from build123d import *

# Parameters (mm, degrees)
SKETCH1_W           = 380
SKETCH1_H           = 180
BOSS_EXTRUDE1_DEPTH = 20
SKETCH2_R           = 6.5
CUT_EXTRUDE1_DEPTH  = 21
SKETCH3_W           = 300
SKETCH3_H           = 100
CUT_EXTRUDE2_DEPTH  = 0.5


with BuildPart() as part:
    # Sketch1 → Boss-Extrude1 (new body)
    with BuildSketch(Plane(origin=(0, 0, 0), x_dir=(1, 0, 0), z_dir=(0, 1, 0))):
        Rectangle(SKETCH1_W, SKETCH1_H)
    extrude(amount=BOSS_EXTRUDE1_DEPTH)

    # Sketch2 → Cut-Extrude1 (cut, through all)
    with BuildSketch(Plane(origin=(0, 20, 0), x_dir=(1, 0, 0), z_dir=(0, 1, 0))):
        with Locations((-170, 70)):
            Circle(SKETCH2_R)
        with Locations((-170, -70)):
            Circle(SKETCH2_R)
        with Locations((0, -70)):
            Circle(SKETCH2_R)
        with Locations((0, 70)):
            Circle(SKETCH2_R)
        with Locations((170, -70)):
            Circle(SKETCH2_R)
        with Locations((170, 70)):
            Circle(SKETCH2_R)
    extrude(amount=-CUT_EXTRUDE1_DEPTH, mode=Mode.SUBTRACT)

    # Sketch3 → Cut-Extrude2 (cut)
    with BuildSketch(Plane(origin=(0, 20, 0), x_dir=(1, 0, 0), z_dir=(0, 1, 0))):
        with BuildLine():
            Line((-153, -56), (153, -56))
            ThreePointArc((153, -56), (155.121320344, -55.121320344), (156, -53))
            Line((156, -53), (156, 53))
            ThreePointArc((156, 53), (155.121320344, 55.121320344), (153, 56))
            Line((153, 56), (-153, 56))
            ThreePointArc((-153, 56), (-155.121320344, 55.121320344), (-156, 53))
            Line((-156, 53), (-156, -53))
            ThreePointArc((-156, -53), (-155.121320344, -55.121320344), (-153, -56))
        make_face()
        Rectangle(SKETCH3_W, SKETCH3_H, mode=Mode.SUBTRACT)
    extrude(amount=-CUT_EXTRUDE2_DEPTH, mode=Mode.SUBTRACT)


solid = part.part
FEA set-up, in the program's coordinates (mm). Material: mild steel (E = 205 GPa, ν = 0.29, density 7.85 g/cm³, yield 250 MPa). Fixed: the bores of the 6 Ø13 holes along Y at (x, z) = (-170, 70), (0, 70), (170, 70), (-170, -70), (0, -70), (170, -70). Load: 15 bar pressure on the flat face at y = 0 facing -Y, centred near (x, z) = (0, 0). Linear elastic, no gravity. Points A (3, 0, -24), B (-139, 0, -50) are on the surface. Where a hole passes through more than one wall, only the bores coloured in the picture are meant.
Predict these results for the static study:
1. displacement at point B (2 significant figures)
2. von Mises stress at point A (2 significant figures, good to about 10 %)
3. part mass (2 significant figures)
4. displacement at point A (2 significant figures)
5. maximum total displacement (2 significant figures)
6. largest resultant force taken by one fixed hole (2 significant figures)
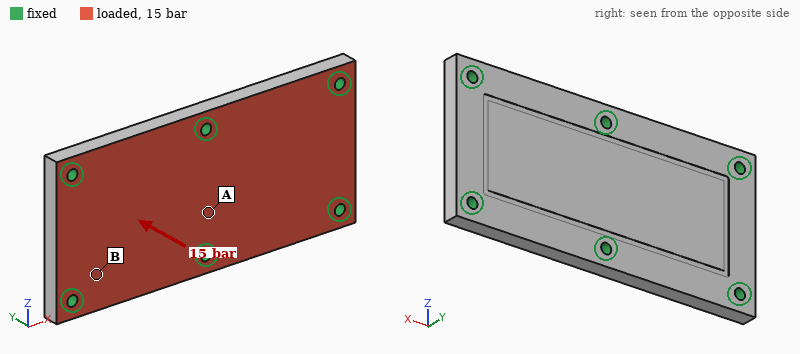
22 µm
36 MPa
11 kg
25 µm
46 µm
24 kN
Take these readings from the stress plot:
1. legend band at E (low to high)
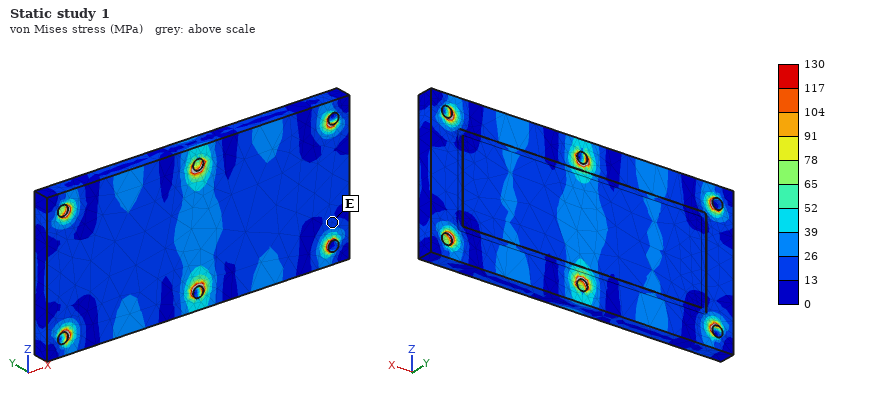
13 to 26 MPa
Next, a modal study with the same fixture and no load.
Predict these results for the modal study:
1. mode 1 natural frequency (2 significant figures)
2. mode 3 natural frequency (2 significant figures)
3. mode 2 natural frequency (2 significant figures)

2600 Hz
3800 Hz
2700 Hz
